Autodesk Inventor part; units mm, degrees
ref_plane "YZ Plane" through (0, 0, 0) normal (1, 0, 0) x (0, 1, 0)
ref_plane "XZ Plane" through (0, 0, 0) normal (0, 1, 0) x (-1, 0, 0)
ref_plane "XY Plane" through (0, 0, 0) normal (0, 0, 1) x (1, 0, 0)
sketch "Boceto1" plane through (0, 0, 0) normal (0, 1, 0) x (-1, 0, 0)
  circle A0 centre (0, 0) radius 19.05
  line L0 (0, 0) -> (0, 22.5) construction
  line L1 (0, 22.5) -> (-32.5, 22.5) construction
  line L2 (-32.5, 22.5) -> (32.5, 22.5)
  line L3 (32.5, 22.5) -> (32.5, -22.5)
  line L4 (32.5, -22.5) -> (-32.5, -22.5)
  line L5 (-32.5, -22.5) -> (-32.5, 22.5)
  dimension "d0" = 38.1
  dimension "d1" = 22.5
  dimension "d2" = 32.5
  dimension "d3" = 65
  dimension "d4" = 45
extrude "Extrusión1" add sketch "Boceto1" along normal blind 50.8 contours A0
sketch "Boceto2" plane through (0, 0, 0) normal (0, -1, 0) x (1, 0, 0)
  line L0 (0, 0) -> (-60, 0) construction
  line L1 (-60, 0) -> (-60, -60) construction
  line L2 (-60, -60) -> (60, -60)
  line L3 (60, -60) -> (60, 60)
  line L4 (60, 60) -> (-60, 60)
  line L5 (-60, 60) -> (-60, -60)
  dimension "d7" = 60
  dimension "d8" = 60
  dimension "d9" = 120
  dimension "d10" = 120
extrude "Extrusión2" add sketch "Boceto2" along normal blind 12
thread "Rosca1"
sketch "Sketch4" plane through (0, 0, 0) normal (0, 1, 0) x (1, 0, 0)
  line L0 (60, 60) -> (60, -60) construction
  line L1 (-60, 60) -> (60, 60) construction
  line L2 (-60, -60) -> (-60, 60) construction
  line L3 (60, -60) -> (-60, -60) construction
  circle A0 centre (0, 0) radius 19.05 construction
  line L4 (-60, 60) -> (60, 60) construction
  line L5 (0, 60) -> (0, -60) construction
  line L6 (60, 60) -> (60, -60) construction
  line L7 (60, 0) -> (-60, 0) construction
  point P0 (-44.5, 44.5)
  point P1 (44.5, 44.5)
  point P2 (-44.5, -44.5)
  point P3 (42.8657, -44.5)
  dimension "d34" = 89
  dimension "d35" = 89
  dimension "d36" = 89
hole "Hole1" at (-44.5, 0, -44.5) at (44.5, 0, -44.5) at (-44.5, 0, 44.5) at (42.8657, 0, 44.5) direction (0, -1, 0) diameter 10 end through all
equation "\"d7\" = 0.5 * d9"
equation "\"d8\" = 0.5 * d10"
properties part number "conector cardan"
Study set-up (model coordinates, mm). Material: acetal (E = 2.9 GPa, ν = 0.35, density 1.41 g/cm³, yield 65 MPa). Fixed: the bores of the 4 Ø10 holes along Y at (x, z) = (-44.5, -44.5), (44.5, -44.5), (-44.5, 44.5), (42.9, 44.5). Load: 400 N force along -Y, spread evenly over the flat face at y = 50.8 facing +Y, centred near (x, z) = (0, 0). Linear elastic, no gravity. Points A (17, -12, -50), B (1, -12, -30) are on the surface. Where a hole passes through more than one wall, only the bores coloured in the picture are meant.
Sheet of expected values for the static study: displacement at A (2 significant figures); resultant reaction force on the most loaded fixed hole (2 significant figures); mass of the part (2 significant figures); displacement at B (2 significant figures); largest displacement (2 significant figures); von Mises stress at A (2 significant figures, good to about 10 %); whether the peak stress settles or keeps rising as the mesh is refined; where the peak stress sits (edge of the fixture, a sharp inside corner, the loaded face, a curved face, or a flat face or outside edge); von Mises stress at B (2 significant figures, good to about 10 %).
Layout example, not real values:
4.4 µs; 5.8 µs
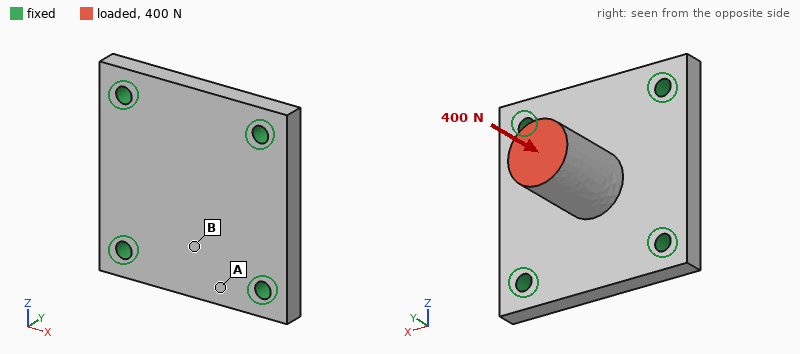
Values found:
14 µm; 100 N; 320 g; 42 µm; 62 µm; 0.47 MPa; keeps rising; edge of the fixture; 0.96 MPa
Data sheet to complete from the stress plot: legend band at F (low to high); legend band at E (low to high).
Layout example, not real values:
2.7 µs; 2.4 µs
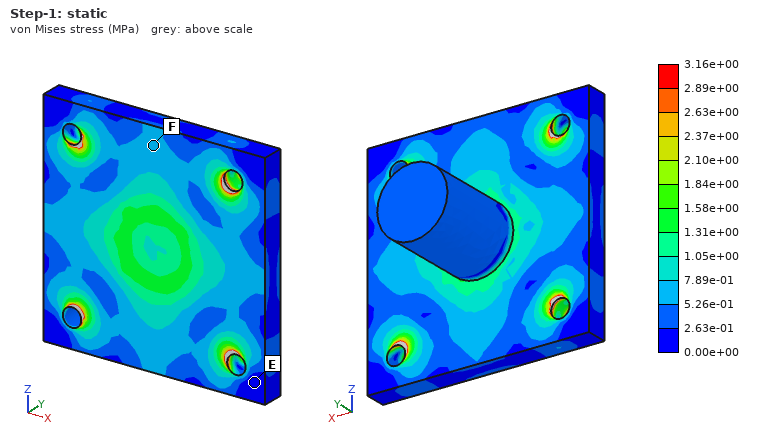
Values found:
5.26e-01 to 7.89e-01 MPa; 0.00e+00 to 2.63e-01 MPa
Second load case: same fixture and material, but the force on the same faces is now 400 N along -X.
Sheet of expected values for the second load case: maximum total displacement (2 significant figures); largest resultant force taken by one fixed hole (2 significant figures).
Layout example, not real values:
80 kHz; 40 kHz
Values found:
0.28 mm; 190 N
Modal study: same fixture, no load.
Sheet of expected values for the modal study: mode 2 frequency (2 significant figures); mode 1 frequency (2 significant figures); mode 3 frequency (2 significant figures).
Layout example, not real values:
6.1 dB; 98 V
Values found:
1100 Hz; 1100 Hz; 1100 Hz
